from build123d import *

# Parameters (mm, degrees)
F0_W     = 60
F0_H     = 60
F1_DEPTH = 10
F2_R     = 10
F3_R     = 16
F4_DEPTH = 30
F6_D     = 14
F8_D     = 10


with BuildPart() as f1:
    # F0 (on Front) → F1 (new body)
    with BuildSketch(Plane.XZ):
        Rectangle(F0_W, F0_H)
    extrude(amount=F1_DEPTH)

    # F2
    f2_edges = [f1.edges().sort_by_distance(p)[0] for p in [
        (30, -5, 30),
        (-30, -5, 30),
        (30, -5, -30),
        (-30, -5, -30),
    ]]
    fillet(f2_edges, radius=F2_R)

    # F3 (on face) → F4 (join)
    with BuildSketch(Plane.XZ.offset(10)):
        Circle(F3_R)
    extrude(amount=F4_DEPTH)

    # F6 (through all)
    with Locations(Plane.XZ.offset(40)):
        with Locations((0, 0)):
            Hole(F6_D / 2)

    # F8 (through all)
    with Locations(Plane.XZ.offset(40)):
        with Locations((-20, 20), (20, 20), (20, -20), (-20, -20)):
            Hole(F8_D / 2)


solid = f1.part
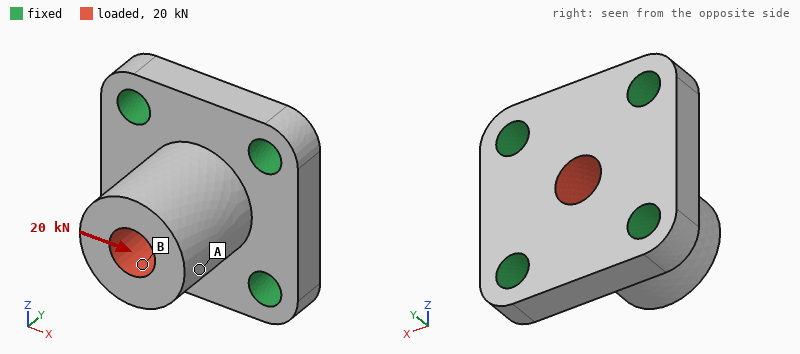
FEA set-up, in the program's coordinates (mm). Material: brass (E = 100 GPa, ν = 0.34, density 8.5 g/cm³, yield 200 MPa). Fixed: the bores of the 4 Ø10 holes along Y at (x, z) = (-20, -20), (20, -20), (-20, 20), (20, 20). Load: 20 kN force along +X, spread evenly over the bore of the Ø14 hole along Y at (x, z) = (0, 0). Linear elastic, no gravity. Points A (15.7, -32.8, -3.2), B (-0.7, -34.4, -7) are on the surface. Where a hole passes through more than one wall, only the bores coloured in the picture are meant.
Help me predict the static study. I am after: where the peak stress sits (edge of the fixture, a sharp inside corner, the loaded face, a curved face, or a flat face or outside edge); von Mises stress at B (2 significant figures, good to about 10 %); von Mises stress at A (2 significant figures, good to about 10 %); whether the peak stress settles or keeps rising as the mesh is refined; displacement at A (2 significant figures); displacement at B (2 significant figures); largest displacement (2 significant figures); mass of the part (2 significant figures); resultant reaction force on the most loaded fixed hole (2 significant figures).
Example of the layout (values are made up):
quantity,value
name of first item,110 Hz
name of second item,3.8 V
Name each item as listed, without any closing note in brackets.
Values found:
quantity,value
where the peak stress sits,edge of the fixture
von Mises stress at B,34 MPa
von Mises stress at A,12 MPa
whether the peak stress settles or keeps rising as the mesh is refined,keeps rising
displacement at A,49 µm
displacement at B,47 µm
largest displacement,59 µm
mass of the part,420 g
resultant reaction force on the most loaded fixed hole,7.0 kN
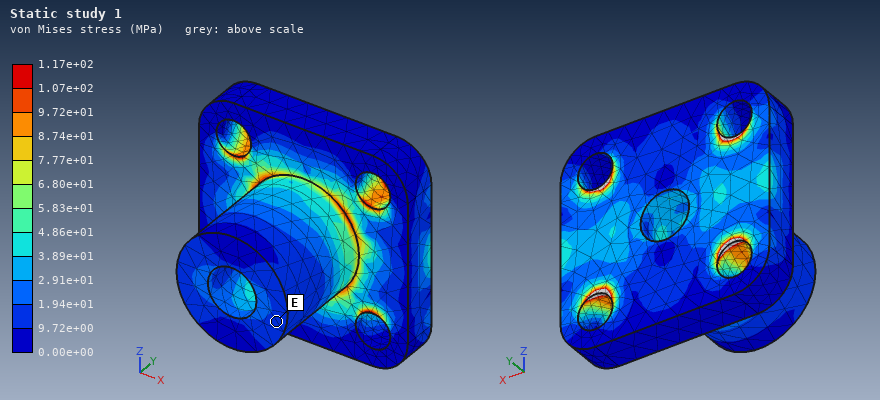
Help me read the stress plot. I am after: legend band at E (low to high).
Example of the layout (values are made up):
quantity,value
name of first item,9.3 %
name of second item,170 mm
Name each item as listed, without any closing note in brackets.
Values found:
quantity,value
legend band at E,9.72e+00 to 1.94e+01 MPa
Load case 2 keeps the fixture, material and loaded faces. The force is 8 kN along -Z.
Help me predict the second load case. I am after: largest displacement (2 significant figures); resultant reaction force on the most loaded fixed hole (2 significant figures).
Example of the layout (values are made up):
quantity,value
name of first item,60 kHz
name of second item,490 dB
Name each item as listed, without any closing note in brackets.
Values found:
quantity,value
largest displacement,23 µm
resultant reaction force on the most loaded fixed hole,2.8 kN
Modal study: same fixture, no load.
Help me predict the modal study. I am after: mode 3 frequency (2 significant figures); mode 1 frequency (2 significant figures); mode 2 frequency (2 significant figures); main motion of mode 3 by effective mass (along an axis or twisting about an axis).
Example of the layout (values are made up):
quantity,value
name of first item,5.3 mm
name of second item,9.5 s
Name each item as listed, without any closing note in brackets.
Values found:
quantity,value
mode 3 frequency,11 kHz
mode 1 frequency,7300 Hz
mode 2 frequency,7300 Hz
main motion of mode 3 by effective mass,along Y
